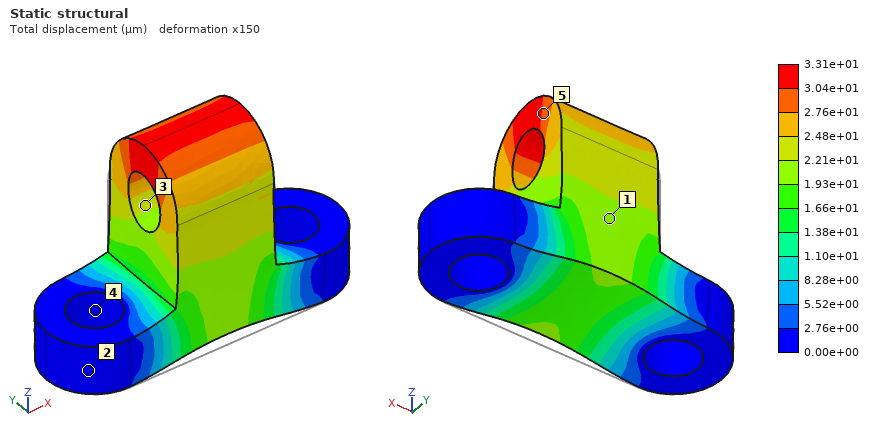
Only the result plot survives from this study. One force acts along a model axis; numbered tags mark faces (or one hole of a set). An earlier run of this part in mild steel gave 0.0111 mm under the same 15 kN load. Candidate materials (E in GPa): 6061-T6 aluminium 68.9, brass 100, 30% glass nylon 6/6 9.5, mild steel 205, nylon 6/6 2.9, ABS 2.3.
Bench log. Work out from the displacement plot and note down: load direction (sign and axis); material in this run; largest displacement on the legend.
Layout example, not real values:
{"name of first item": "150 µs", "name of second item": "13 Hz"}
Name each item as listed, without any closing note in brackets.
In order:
{"load direction": "+Z", "material in this run": "6061-T6 aluminium", "largest displacement on the legend": "3.31e+01 µm"}
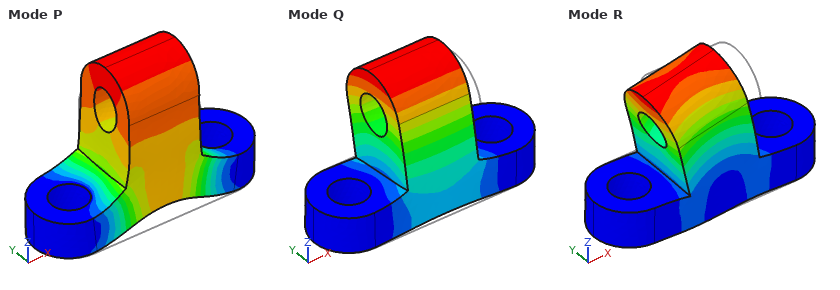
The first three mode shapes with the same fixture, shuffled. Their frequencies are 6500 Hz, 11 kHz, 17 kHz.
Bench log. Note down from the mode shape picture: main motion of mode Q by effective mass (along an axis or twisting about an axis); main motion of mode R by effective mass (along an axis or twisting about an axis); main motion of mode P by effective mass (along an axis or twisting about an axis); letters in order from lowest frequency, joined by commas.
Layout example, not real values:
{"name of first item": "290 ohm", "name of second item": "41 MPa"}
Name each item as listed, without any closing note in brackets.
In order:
{"main motion of mode Q by effective mass": "along Y", "main motion of mode R by effective mass": "along X", "main motion of mode P by effective mass": "along Z", "letters in order from lowest frequency, joined by commas": "Q, R, P"}
